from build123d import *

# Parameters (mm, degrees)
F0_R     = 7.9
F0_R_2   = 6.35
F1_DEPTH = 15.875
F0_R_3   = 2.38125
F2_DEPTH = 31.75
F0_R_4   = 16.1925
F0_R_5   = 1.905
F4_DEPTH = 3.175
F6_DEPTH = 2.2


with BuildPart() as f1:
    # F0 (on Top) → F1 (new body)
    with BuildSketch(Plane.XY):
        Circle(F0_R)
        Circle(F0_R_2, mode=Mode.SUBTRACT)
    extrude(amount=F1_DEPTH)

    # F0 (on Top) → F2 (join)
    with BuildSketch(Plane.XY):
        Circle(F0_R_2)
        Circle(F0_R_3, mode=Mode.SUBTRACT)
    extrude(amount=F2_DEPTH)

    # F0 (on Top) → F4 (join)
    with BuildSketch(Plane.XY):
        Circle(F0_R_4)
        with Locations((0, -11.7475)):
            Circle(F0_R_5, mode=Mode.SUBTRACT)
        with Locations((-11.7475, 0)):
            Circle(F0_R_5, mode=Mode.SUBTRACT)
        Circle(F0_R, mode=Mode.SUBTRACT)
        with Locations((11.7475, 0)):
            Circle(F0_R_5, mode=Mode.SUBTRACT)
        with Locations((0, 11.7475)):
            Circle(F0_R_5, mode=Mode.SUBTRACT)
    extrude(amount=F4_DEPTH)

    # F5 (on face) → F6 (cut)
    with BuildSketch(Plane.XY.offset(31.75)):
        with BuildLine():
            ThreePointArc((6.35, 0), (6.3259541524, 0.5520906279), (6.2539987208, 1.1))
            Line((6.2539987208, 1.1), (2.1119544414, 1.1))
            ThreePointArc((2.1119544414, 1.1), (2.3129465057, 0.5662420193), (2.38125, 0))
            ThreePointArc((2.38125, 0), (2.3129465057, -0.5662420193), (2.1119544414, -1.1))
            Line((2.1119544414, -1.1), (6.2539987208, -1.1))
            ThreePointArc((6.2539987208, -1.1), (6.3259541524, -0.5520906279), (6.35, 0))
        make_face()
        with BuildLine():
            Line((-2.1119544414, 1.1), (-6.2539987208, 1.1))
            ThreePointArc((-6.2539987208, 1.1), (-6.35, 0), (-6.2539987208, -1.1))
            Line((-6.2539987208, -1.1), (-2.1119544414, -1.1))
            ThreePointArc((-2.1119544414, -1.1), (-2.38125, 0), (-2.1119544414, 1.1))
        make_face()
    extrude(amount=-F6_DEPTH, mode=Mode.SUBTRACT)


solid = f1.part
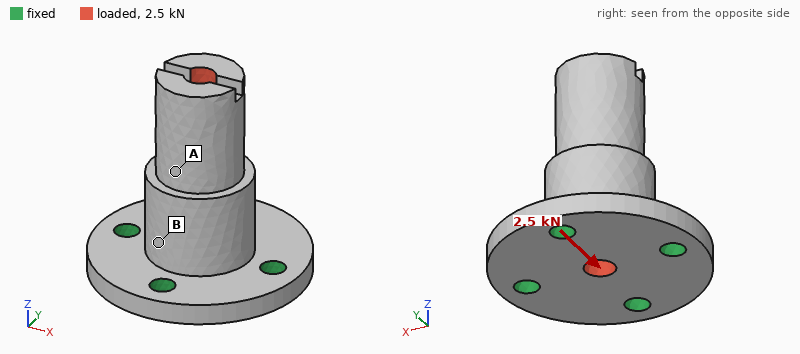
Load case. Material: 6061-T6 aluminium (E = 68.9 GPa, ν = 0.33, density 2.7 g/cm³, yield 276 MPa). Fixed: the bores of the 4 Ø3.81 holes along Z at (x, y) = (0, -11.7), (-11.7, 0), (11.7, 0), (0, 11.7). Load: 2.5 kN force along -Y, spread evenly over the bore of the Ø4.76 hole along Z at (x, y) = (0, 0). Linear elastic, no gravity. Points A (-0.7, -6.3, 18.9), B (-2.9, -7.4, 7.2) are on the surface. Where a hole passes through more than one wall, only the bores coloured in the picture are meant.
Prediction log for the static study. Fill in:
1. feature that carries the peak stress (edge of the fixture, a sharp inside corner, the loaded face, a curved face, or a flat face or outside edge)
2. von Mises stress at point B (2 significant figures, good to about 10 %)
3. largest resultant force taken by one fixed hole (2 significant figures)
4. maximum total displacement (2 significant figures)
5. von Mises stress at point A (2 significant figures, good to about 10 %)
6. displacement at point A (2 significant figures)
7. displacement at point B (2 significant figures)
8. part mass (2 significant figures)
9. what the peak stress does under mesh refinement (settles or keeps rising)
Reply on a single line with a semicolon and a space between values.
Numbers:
edge of the fixture; 61 MPa; 1.9 kN; 0.10 mm; 30 MPa; 0.055 mm; 0.022 mm; 17 g; keeps rising
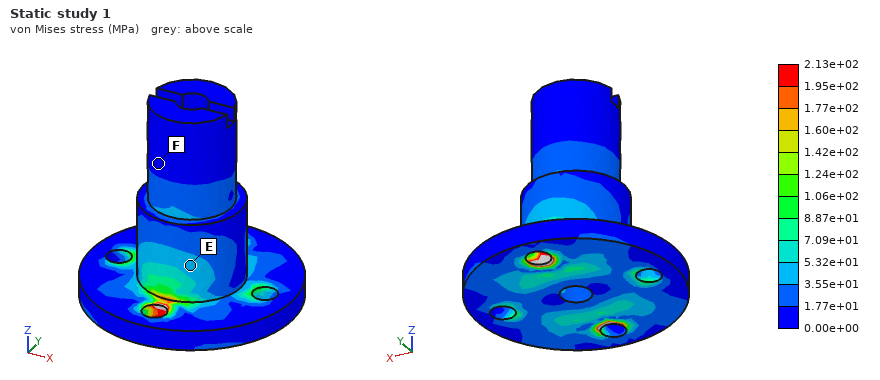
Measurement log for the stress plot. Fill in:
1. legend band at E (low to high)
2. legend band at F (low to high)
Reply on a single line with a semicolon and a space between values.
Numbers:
3.55e+01 to 5.32e+01 MPa; 0.00e+00 to 1.77e+01 MPa
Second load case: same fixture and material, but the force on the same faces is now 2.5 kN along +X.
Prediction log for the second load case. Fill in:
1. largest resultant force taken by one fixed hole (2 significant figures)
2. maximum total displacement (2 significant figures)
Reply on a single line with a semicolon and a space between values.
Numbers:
1.9 kN; 0.10 mm
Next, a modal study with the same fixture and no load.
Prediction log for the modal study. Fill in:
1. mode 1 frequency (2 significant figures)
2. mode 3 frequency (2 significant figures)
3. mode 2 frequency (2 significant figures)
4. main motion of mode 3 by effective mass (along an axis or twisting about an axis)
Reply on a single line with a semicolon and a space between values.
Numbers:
9800 Hz; 26 kHz; 9800 Hz; along Z
